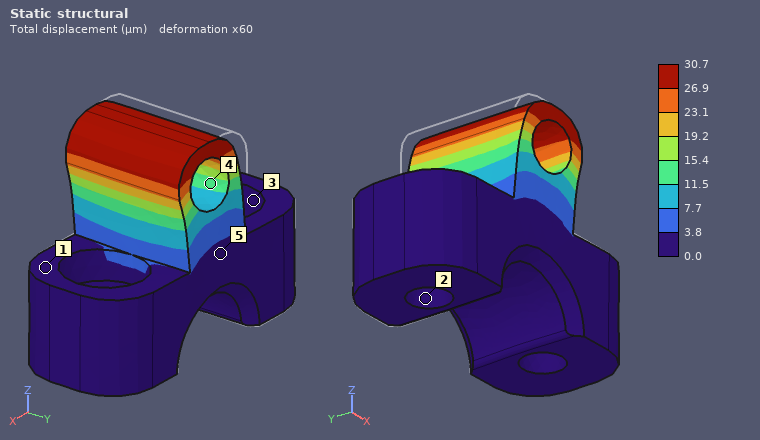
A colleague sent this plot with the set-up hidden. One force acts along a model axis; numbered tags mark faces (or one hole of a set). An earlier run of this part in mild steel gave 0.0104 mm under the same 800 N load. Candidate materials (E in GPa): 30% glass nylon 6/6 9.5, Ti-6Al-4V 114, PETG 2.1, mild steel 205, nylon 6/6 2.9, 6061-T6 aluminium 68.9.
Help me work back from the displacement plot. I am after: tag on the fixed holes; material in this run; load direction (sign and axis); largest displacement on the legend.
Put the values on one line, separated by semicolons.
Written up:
2; 6061-T6 aluminium; +X; 30.7 µm
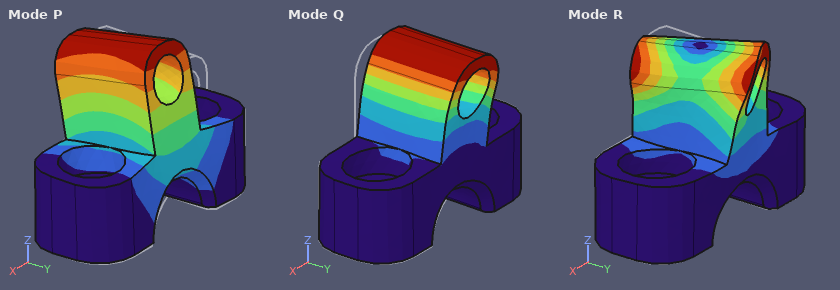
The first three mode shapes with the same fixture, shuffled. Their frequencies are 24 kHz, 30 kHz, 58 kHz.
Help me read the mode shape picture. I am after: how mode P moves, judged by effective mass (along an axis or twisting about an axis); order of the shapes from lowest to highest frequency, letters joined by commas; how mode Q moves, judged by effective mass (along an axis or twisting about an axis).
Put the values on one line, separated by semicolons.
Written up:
along Y; P, Q, R; along X
